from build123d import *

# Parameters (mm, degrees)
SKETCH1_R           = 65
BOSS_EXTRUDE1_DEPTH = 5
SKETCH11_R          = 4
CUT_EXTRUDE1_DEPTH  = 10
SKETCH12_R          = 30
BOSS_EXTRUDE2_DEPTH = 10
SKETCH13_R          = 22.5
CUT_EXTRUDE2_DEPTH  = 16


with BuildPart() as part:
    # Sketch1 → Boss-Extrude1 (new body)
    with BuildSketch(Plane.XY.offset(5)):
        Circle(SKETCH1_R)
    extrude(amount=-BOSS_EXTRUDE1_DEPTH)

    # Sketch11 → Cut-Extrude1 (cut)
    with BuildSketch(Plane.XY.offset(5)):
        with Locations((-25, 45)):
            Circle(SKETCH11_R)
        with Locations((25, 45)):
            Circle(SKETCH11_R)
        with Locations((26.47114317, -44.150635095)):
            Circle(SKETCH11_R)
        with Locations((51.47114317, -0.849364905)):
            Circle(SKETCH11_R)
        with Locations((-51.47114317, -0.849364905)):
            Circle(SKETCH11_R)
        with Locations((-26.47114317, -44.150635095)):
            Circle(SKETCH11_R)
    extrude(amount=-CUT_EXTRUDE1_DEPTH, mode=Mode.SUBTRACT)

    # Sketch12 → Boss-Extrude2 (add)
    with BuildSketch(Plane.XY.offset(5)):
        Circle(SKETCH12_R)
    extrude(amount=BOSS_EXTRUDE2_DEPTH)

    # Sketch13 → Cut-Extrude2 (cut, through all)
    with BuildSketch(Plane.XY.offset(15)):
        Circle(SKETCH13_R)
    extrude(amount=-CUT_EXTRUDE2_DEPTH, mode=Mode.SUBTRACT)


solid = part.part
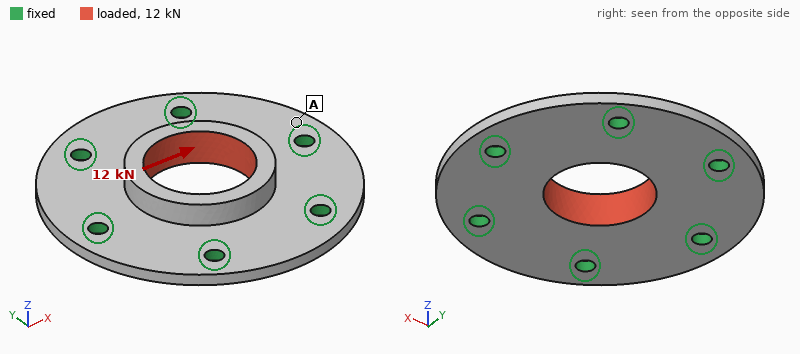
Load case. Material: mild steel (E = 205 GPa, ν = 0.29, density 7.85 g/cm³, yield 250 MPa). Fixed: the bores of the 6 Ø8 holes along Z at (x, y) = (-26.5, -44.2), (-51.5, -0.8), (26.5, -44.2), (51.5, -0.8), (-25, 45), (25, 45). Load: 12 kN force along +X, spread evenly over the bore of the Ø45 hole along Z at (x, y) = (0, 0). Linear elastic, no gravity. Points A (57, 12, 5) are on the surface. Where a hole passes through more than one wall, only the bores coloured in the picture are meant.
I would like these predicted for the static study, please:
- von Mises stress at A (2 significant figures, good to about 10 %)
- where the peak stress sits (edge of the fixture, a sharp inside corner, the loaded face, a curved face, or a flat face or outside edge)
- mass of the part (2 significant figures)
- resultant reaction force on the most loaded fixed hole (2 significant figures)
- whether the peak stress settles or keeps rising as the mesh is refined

5.5 MPa
edge of the fixture
540 g
2.8 kN
keeps rising
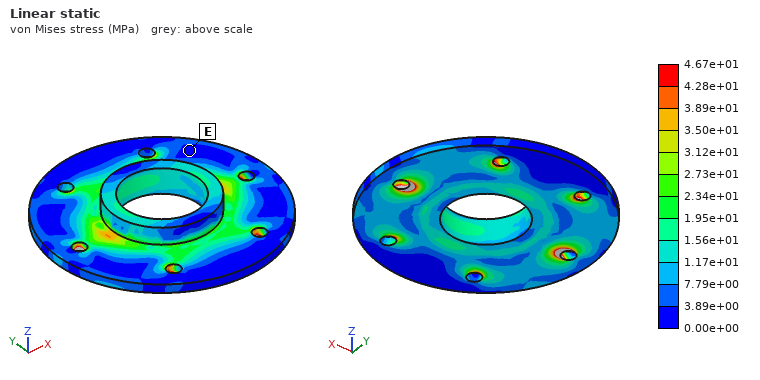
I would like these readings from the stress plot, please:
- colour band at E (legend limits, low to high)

0.00e+00 to 3.89e+00 MPa
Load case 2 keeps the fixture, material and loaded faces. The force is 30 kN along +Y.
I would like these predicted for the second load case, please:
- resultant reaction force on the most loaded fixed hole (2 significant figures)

6.2 kN
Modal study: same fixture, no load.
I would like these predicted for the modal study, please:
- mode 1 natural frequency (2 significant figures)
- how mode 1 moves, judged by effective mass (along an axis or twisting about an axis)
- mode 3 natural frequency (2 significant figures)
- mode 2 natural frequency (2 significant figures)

6100 Hz
along Z
7900 Hz
7900 Hz
